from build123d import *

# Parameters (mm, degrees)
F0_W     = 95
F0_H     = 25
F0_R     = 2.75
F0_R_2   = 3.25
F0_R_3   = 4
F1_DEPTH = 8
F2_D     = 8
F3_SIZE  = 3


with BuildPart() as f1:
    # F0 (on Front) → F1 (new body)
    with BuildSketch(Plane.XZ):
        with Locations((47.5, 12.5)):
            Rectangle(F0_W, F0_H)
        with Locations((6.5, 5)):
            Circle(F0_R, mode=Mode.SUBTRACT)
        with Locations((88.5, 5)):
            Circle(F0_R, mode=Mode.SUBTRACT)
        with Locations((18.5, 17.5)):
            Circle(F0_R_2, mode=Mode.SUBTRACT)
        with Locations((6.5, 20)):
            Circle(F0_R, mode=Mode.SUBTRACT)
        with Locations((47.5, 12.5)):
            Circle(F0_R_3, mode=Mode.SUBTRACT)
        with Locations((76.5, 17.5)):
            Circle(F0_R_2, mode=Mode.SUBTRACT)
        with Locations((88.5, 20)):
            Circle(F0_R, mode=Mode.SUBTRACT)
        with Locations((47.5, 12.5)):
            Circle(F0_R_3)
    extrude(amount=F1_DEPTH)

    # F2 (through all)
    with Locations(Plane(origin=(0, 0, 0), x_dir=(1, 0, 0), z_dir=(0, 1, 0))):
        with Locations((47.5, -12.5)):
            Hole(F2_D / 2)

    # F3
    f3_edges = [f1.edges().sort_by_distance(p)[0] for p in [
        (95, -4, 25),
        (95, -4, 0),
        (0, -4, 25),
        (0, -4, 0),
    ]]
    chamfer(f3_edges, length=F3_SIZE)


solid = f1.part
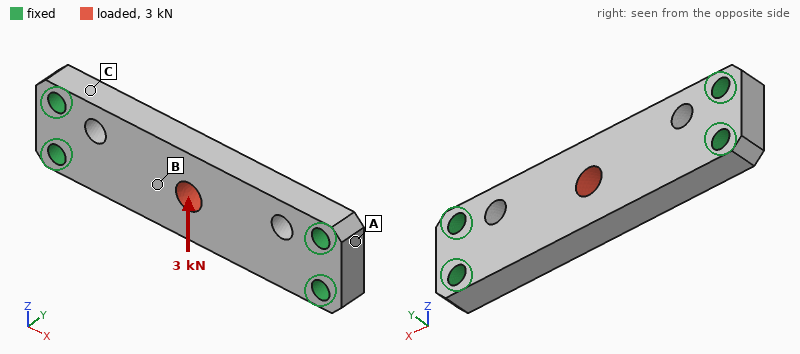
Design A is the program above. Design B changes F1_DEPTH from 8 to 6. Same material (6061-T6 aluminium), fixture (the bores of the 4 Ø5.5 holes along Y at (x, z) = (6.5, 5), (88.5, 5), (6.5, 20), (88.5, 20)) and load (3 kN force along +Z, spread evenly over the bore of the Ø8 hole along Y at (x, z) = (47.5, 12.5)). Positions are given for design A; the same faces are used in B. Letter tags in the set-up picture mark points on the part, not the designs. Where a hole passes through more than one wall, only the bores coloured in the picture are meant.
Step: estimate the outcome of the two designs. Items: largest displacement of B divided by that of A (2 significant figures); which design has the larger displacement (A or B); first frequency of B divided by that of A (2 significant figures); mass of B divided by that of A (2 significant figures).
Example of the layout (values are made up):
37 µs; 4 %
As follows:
1.3; B; 0.78; 0.75
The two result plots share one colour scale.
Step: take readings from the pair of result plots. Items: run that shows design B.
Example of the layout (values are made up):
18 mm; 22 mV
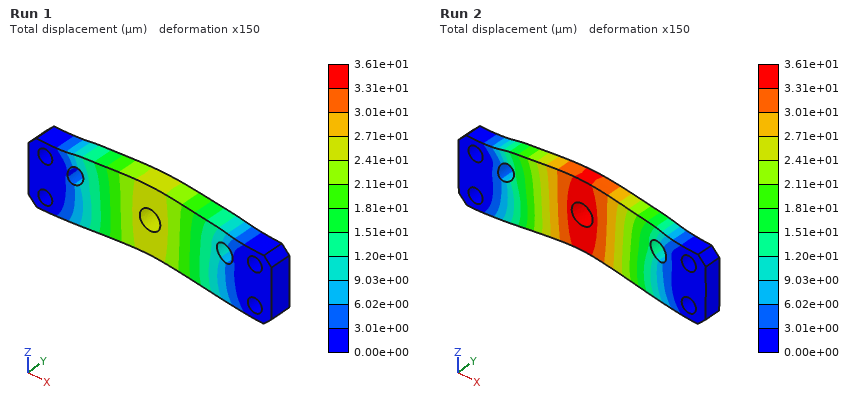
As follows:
Run 2
